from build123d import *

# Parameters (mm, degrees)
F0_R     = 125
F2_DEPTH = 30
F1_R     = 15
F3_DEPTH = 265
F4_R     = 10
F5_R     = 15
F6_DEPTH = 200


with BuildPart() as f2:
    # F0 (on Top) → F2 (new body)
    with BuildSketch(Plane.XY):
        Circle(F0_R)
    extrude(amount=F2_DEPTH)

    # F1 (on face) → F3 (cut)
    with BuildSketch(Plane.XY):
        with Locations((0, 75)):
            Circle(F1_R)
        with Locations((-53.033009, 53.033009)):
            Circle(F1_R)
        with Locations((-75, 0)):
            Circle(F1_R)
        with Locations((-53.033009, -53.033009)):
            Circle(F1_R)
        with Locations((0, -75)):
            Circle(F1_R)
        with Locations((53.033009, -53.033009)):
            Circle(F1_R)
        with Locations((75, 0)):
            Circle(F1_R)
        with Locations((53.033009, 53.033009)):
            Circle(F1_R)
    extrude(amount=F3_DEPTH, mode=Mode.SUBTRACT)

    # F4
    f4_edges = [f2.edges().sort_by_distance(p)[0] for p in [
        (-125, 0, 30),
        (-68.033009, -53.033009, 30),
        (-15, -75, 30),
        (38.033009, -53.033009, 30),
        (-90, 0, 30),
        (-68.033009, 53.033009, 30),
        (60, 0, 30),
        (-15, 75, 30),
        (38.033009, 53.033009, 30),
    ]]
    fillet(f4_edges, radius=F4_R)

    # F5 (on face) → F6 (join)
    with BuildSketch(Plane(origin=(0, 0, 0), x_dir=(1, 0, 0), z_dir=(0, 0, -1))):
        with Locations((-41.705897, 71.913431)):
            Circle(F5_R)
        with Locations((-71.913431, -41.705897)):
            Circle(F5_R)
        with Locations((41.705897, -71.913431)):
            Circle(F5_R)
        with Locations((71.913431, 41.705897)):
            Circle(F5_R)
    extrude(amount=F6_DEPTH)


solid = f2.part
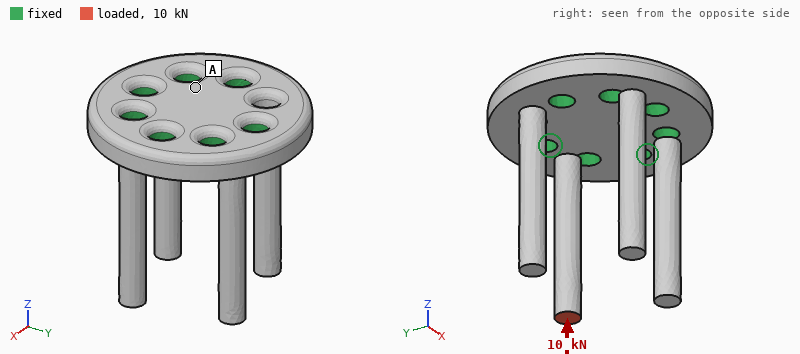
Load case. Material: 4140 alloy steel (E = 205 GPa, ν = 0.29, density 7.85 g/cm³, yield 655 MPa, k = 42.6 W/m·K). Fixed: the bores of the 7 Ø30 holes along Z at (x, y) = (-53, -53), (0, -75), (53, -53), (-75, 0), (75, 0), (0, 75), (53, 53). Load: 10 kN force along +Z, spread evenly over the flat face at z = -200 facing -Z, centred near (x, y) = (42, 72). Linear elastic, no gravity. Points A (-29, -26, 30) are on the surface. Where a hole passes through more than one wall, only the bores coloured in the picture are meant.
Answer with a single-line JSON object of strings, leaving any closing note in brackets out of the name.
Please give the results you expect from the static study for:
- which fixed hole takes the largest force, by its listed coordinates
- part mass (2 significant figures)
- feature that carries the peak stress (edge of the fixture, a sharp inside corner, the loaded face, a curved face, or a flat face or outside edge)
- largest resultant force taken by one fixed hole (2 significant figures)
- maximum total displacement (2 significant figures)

{"which fixed hole takes the largest force, by its listed coordinates": "(53, 53)", "part mass": "14 kg", "feature that carries the peak stress": "a curved face", "largest resultant force taken by one fixed hole": "7.9 kN", "maximum total displacement": "16 µm"}
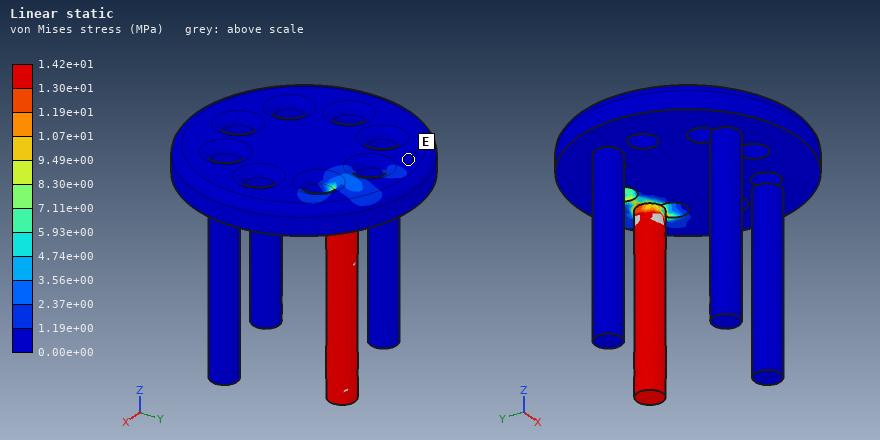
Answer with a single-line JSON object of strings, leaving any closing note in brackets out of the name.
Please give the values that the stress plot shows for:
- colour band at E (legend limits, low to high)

{"colour band at E": "0.00e+00 to 1.19e+00 MPa"}
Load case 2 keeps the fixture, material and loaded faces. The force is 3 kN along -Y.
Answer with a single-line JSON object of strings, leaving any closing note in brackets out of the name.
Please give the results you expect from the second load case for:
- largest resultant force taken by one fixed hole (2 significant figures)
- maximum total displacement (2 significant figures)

{"largest resultant force taken by one fixed hole": "10 kN", "maximum total displacement": "1.1 mm"}
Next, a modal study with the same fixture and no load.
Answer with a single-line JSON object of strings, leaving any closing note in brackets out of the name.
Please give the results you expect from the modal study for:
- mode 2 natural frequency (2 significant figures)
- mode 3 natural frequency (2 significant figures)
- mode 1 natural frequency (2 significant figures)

{"mode 2 natural frequency": "470 Hz", "mode 3 natural frequency": "480 Hz", "mode 1 natural frequency": "450 Hz"}
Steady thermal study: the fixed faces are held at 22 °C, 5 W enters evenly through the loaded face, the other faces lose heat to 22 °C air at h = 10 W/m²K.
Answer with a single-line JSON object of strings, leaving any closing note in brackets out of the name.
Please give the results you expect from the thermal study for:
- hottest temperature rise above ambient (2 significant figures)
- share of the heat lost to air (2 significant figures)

{"hottest temperature rise above ambient": "24 K", "share of the heat lost to air": "43 %"}
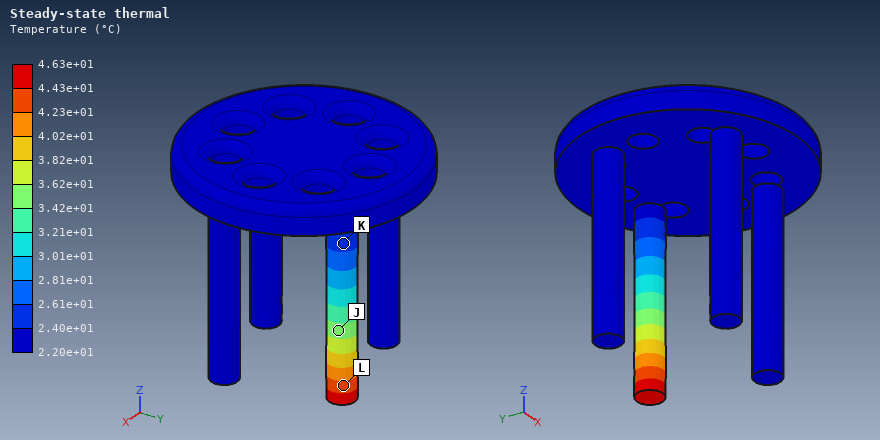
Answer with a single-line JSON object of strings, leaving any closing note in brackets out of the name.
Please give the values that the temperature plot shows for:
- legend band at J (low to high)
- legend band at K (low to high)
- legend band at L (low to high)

{"legend band at J": "3.42e+01 to 3.62e+01 °C", "legend band at K": "2.40e+01 to 2.61e+01 °C", "legend band at L": "4.23e+01 to 4.43e+01 °C"}
